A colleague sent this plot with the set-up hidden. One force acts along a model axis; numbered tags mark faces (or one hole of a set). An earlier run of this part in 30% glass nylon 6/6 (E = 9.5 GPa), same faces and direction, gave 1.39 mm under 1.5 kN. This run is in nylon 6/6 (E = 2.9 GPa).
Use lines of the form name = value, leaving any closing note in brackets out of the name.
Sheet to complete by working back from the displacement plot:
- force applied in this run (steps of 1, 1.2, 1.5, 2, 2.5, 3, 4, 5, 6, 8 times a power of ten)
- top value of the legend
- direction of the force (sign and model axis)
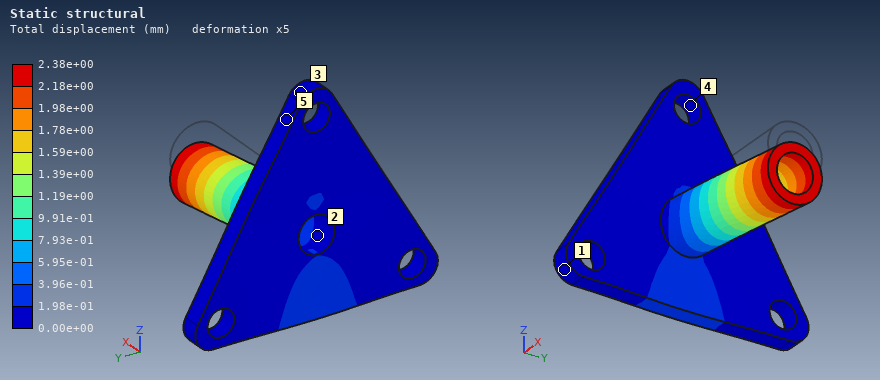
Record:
force applied in this run = 800 N
top value of the legend = 2.38e+00 mm
direction of the force = -Z
